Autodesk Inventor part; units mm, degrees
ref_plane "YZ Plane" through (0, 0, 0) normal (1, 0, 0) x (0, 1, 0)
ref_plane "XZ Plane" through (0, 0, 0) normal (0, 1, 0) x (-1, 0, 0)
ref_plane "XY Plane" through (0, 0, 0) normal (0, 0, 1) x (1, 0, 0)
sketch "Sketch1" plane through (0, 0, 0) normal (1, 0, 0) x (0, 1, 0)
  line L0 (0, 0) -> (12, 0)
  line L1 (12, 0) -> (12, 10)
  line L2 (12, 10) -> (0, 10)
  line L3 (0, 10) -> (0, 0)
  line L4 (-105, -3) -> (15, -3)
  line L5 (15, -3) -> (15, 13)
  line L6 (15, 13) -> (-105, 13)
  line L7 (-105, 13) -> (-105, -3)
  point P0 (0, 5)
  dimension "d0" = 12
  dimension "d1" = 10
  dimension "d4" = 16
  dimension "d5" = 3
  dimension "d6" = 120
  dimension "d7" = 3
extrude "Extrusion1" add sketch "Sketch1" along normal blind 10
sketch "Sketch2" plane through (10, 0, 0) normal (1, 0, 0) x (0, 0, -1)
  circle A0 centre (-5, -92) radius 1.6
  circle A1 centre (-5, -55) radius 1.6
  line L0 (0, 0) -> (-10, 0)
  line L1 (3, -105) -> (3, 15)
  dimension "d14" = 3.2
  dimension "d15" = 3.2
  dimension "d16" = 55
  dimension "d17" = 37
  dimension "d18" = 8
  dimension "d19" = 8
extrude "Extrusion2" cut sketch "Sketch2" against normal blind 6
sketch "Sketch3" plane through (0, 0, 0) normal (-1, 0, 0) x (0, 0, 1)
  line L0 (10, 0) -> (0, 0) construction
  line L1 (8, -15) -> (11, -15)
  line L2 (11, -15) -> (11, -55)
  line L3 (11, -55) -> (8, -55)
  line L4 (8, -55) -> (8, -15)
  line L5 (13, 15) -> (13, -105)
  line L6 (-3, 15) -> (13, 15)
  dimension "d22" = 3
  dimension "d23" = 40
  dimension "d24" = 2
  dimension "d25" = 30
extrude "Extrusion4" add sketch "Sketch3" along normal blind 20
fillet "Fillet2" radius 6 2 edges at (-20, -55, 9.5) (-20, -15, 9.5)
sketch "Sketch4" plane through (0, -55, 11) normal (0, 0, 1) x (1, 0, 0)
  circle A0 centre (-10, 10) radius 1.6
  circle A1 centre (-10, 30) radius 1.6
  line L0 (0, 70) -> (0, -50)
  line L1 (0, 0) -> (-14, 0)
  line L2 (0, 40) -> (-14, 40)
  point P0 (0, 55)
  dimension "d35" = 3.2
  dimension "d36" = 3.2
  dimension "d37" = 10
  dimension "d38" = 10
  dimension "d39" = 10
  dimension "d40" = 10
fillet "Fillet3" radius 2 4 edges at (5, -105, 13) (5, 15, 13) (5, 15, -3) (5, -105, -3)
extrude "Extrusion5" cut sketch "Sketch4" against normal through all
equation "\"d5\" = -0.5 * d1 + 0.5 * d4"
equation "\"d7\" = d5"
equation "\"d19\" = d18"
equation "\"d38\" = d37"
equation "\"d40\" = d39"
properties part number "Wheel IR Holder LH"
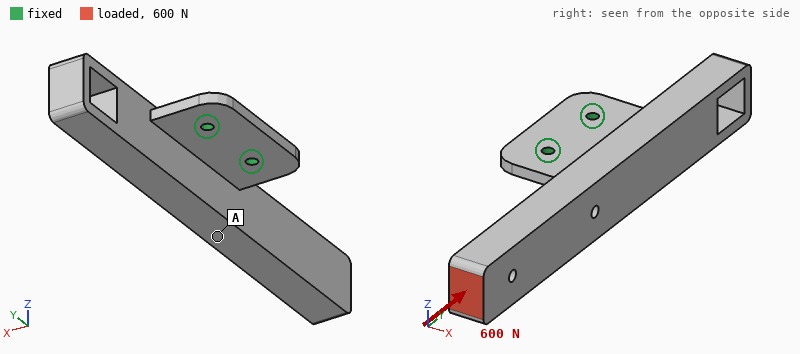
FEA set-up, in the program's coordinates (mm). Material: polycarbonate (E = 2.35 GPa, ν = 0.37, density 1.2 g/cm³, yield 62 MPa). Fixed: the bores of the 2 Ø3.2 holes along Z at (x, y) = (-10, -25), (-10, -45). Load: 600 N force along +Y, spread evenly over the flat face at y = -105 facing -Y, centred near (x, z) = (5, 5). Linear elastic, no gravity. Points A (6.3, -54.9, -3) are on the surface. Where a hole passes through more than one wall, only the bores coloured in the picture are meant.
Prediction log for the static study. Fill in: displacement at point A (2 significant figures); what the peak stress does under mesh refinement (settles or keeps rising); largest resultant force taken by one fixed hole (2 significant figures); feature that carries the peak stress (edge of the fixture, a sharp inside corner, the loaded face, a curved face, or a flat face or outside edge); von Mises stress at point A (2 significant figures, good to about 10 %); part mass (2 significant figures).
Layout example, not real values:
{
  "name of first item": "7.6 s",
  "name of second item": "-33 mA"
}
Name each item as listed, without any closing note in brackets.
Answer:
{
  "displacement at point A": "0.51 mm",
  "what the peak stress does under mesh refinement": "keeps rising",
  "largest resultant force taken by one fixed hole": "520 N",
  "feature that carries the peak stress": "edge of the fixture",
  "von Mises stress at point A": "4.2 MPa",
  "part mass": "24 g"
}
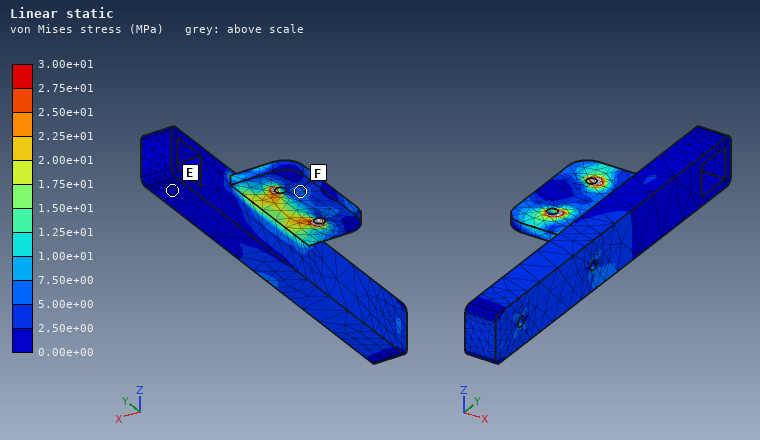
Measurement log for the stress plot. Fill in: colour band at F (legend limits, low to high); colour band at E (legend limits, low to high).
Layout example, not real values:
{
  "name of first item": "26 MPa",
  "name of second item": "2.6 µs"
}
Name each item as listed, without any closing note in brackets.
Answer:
{
  "colour band at F": "5.00e+00 to 7.50e+00 MPa",
  "colour band at E": "0.00e+00 to 2.50e+00 MPa"
}
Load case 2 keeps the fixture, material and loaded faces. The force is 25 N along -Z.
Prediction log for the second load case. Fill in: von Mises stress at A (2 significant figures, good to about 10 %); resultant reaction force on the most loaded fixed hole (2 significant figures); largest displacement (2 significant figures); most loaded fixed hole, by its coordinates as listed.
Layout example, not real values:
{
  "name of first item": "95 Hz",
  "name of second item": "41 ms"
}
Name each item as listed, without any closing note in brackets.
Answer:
{
  "von Mises stress at A": "3.1 MPa",
  "resultant reaction force on the most loaded fixed hole": "84 N",
  "largest displacement": "1.3 mm",
  "most loaded fixed hole, by its coordinates as listed": "(-10, -45)"
}
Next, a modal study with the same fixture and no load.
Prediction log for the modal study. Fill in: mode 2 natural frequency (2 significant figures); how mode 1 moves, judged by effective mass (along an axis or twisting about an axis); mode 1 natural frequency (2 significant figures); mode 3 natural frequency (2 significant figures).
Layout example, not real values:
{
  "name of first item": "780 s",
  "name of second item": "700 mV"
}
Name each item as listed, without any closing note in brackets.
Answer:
{
  "mode 2 natural frequency": "450 Hz",
  "how mode 1 moves, judged by effective mass": "along Z",
  "mode 1 natural frequency": "310 Hz",
  "mode 3 natural frequency": "590 Hz"
}
